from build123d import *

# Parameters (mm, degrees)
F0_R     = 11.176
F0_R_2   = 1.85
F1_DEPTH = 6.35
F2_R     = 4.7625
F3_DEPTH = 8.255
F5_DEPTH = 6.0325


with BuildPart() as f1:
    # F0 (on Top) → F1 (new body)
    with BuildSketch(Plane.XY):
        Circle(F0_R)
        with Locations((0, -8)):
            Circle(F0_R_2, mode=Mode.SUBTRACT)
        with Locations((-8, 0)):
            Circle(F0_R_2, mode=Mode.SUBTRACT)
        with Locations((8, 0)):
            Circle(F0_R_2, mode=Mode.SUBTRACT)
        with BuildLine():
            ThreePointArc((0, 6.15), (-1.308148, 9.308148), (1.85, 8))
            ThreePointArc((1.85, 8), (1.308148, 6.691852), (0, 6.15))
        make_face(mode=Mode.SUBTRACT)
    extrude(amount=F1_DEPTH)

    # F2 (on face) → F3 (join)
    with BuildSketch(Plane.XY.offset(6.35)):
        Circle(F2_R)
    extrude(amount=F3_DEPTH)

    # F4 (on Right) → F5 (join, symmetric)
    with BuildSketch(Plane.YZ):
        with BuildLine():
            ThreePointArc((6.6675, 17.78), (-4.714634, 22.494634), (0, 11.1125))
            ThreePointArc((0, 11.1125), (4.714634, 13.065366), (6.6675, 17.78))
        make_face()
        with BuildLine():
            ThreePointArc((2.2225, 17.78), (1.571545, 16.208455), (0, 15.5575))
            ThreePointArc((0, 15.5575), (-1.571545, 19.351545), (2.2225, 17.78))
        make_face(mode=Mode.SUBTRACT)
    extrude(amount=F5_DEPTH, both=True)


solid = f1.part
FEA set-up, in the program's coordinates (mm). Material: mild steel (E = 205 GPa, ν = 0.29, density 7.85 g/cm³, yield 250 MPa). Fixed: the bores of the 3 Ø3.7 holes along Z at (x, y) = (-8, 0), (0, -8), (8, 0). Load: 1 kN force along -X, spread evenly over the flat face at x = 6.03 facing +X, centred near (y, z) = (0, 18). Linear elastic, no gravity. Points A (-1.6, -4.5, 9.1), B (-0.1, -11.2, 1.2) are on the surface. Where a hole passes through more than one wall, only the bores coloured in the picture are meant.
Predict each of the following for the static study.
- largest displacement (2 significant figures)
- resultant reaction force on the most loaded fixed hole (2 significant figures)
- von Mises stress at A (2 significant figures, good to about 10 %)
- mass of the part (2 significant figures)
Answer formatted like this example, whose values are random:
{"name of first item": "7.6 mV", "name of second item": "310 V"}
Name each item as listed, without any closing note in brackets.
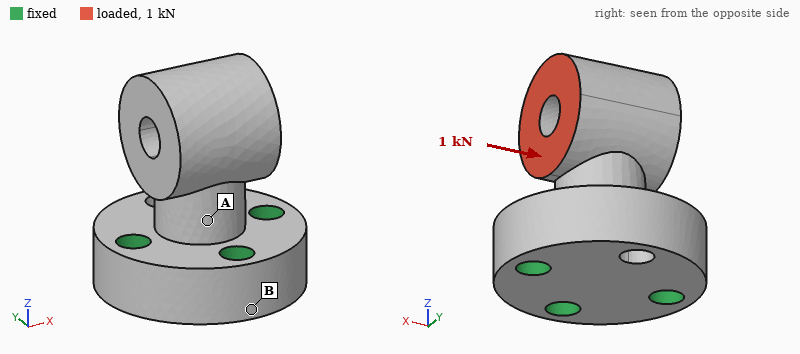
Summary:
{"largest displacement": "21 µm", "resultant reaction force on the most loaded fixed hole": "1.1 kN", "von Mises stress at A": "42 MPa", "mass of the part": "32 g"}
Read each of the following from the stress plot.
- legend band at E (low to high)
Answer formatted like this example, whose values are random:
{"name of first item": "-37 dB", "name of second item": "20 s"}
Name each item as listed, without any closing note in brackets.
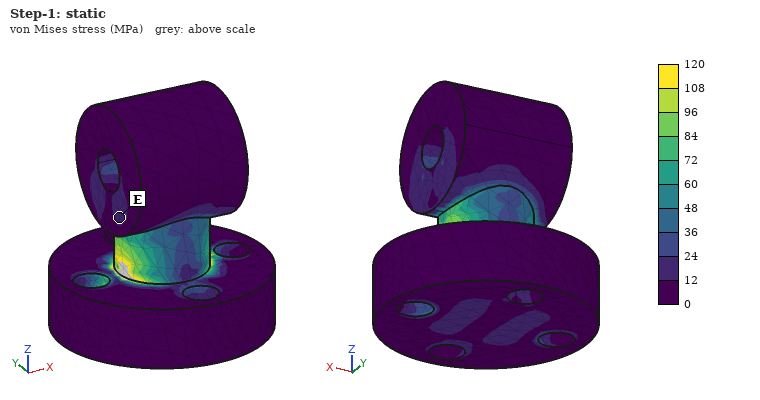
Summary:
{"legend band at E": "12 to 24 MPa"}
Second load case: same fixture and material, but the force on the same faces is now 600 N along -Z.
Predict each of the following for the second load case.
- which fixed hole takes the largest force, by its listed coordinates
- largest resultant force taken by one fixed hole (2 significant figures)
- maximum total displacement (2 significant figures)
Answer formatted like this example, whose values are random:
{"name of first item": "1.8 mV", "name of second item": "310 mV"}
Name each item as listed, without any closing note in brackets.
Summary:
{"which fixed hole takes the largest force, by its listed coordinates": "(8, 0)", "largest resultant force taken by one fixed hole": "490 N", "maximum total displacement": "8.3 µm"}
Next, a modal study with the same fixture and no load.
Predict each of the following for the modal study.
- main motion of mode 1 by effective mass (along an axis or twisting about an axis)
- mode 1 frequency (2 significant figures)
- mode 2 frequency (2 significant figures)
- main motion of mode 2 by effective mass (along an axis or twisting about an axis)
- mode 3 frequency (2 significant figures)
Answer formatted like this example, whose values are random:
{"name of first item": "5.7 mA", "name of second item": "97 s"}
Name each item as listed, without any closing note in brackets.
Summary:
{"main motion of mode 1 by effective mass": "along Y", "mode 1 frequency": "11 kHz", "mode 2 frequency": "12 kHz", "main motion of mode 2 by effective mass": "along X", "mode 3 frequency": "25 kHz"}
